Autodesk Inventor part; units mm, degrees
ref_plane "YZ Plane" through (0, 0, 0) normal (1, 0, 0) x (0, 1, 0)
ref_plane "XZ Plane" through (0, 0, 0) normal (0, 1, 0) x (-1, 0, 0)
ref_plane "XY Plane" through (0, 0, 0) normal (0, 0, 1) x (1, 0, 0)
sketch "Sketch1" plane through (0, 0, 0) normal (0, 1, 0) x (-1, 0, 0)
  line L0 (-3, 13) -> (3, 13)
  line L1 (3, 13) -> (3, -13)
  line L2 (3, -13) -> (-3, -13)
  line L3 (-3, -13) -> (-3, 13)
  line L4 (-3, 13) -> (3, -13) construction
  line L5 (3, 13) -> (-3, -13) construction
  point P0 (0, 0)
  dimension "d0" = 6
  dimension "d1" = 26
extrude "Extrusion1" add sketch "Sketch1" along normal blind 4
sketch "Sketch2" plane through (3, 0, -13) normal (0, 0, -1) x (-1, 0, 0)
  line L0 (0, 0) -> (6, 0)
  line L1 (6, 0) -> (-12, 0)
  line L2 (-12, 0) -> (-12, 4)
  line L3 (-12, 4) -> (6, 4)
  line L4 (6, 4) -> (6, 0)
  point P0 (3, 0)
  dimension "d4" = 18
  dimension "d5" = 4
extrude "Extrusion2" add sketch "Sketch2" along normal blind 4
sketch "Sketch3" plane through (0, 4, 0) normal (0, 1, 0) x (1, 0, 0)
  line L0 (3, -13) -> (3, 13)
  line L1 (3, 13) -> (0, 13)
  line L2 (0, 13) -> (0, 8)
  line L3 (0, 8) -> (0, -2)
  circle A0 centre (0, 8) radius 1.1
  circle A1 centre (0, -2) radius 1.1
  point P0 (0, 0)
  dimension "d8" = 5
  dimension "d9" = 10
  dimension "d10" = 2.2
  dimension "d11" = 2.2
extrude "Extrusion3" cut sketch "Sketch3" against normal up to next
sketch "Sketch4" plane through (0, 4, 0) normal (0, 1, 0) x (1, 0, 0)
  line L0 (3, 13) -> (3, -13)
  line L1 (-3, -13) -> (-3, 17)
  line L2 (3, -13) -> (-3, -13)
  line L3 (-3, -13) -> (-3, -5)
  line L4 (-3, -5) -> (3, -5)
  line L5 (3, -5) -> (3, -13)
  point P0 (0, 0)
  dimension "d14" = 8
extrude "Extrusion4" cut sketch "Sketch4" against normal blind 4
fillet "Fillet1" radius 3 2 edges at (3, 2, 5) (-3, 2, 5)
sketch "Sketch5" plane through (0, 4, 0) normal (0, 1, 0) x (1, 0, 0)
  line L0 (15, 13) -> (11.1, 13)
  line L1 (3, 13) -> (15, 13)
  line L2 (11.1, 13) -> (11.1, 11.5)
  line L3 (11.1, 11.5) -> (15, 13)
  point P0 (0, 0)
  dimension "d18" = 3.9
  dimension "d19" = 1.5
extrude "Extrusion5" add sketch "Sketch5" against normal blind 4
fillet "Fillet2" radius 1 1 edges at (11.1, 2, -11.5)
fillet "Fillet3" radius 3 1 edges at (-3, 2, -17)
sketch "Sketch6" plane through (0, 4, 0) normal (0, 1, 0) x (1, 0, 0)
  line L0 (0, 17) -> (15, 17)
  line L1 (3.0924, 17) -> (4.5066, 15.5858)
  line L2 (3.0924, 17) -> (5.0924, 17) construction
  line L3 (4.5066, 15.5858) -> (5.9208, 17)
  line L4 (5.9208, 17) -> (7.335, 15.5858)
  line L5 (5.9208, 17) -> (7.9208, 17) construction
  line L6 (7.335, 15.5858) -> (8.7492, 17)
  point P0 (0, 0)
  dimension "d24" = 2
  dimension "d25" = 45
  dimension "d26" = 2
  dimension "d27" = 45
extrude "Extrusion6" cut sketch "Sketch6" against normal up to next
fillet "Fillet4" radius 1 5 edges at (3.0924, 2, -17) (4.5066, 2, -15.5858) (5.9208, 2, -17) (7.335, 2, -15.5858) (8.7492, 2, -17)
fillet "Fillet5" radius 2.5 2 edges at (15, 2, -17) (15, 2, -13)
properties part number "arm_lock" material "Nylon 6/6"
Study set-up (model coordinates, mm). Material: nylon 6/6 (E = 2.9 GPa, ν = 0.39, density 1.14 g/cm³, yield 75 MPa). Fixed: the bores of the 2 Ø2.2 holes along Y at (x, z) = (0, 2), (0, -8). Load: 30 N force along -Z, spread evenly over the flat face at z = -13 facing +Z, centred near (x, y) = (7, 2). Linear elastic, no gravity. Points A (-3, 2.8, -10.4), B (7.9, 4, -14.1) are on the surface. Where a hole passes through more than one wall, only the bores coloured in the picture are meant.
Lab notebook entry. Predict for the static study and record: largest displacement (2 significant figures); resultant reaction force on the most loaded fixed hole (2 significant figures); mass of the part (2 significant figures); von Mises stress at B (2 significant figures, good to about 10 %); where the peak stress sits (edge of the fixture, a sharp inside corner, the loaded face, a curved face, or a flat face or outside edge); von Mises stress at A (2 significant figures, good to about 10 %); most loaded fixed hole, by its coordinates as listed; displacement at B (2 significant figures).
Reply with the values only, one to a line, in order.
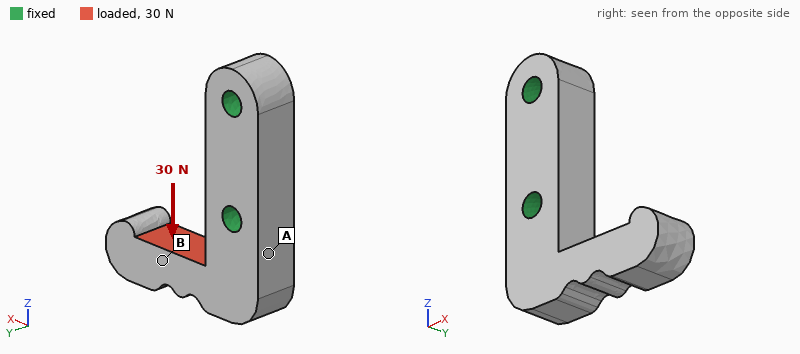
0.27 mm
30 N
0.73 g
3.3 MPa
a curved face
7.8 MPa
(0, -8)
0.12 mm
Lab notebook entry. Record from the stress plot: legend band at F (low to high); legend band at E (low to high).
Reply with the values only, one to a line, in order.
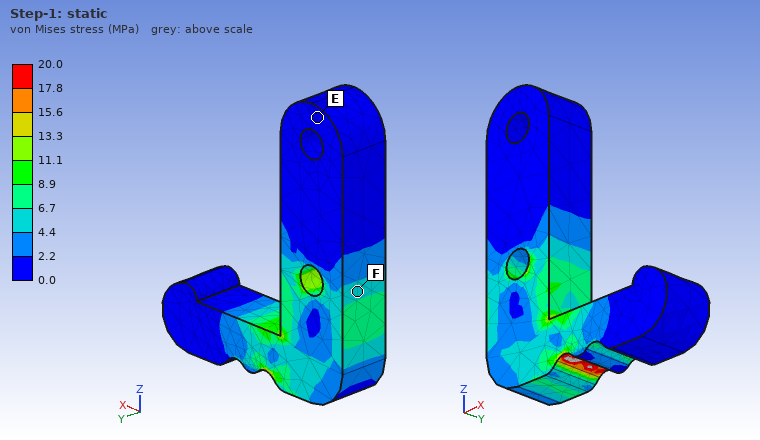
4.4 to 6.7 MPa
0.0 to 2.2 MPa
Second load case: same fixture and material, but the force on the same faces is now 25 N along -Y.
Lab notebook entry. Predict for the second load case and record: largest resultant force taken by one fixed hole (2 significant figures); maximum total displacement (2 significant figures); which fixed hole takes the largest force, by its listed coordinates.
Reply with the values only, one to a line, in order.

26 N
0.30 mm
(0, -8)
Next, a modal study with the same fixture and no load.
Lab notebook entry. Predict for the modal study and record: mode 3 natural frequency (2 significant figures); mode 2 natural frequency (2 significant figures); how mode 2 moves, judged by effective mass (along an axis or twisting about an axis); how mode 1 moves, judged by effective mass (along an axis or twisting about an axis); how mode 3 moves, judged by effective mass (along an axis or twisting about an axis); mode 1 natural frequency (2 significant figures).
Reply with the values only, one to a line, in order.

9900 Hz
3600 Hz
along Z
along Y
along X
3300 Hz
